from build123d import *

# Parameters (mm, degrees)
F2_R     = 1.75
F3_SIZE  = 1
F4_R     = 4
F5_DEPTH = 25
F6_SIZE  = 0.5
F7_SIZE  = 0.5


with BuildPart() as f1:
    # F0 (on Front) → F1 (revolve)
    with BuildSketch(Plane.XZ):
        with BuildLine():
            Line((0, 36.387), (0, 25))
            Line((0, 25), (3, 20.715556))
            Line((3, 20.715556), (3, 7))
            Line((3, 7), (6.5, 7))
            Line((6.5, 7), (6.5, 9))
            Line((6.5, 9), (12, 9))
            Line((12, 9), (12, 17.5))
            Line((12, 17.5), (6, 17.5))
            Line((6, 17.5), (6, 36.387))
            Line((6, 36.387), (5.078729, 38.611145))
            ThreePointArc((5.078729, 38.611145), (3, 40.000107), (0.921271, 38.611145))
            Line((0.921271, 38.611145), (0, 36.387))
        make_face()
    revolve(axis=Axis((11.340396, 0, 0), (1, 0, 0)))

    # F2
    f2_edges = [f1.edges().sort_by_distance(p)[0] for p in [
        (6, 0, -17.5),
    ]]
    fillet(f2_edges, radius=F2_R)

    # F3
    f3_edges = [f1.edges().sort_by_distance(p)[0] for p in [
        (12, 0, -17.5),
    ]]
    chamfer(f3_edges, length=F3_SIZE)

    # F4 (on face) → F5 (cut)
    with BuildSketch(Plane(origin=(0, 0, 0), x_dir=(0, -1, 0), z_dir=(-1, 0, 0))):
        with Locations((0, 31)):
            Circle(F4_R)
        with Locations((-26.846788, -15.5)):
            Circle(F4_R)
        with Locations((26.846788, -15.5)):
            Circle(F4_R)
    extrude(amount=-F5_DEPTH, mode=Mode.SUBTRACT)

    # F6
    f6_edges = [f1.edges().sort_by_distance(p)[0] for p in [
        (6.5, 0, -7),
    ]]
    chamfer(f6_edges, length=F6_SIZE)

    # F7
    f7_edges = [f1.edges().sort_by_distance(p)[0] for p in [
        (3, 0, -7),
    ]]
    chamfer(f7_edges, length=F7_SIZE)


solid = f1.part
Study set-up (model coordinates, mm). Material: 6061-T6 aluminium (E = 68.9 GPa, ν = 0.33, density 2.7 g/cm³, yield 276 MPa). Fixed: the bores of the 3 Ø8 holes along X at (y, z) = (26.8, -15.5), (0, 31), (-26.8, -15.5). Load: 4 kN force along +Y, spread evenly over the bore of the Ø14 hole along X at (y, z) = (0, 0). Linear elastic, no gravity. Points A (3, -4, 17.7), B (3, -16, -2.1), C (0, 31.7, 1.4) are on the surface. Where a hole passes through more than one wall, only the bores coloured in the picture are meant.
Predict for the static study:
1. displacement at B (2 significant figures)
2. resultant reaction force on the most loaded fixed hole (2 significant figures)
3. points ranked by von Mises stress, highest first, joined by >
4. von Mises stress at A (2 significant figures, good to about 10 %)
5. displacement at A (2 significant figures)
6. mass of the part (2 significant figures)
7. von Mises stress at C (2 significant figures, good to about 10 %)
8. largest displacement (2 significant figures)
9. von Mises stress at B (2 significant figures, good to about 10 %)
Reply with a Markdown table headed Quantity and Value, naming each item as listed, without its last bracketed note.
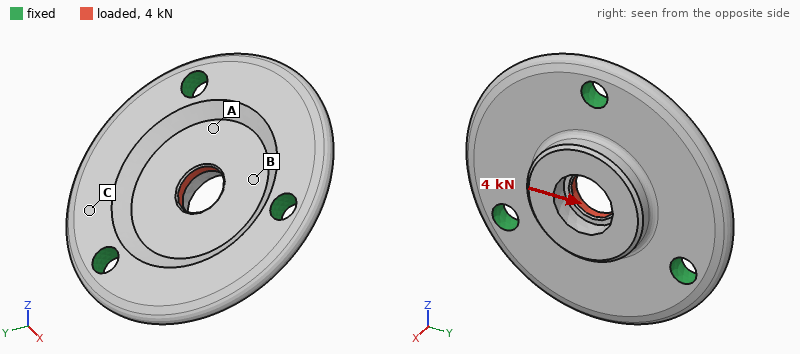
| Quantity | Value |
|---|---|
| displacement at B | 5.3 µm |
| resultant reaction force on the most loaded fixed hole | 1.4 kN |
| points ranked by von Mises stress, highest first, joined by > | B > A > C |
| von Mises stress at A | 13 MPa |
| displacement at A | 3.9 µm |
| mass of the part | 72 g |
| von Mises stress at C | 3.9 MPa |
| largest displacement | 9.1 µm |
| von Mises stress at B | 23 MPa |
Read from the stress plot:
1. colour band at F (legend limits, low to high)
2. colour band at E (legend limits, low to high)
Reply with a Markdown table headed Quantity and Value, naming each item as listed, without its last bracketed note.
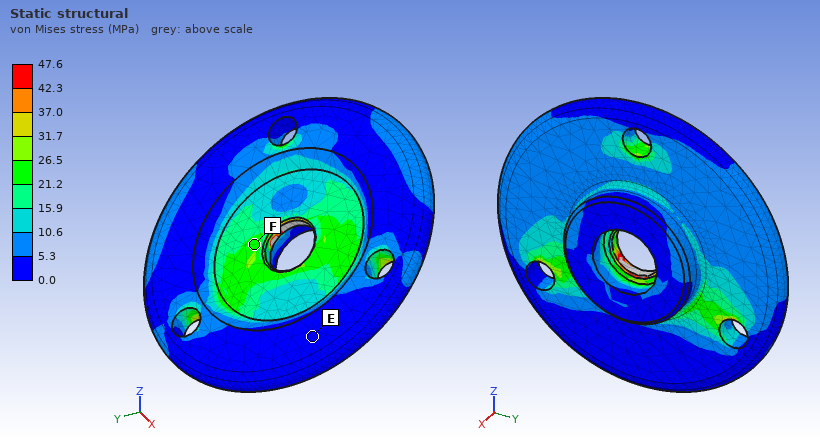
| Quantity | Value |
|---|---|
| colour band at F | 21.2 to 26.5 MPa |
| colour band at E | 0.0 to 5.3 MPa |
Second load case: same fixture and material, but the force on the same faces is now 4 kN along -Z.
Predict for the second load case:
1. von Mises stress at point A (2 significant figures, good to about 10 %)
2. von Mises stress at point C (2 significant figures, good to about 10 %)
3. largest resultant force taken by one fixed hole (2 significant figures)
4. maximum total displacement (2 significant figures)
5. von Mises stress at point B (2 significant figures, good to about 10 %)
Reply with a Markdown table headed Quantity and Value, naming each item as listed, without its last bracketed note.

| Quantity | Value |
|---|---|
| von Mises stress at point A | 25 MPa |
| von Mises stress at point C | 3.4 MPa |
| largest resultant force taken by one fixed hole | 1.4 kN |
| maximum total displacement | 9.2 µm |
| von Mises stress at point B | 12 MPa |
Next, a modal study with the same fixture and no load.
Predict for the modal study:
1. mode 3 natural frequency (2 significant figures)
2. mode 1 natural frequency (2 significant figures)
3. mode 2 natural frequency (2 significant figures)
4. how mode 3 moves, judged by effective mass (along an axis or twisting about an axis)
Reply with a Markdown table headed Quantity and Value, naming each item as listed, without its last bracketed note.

| Quantity | Value |
|---|---|
| mode 3 natural frequency | 7900 Hz |
| mode 1 natural frequency | 7500 Hz |
| mode 2 natural frequency | 7500 Hz |
| how mode 3 moves, judged by effective mass | along X |
